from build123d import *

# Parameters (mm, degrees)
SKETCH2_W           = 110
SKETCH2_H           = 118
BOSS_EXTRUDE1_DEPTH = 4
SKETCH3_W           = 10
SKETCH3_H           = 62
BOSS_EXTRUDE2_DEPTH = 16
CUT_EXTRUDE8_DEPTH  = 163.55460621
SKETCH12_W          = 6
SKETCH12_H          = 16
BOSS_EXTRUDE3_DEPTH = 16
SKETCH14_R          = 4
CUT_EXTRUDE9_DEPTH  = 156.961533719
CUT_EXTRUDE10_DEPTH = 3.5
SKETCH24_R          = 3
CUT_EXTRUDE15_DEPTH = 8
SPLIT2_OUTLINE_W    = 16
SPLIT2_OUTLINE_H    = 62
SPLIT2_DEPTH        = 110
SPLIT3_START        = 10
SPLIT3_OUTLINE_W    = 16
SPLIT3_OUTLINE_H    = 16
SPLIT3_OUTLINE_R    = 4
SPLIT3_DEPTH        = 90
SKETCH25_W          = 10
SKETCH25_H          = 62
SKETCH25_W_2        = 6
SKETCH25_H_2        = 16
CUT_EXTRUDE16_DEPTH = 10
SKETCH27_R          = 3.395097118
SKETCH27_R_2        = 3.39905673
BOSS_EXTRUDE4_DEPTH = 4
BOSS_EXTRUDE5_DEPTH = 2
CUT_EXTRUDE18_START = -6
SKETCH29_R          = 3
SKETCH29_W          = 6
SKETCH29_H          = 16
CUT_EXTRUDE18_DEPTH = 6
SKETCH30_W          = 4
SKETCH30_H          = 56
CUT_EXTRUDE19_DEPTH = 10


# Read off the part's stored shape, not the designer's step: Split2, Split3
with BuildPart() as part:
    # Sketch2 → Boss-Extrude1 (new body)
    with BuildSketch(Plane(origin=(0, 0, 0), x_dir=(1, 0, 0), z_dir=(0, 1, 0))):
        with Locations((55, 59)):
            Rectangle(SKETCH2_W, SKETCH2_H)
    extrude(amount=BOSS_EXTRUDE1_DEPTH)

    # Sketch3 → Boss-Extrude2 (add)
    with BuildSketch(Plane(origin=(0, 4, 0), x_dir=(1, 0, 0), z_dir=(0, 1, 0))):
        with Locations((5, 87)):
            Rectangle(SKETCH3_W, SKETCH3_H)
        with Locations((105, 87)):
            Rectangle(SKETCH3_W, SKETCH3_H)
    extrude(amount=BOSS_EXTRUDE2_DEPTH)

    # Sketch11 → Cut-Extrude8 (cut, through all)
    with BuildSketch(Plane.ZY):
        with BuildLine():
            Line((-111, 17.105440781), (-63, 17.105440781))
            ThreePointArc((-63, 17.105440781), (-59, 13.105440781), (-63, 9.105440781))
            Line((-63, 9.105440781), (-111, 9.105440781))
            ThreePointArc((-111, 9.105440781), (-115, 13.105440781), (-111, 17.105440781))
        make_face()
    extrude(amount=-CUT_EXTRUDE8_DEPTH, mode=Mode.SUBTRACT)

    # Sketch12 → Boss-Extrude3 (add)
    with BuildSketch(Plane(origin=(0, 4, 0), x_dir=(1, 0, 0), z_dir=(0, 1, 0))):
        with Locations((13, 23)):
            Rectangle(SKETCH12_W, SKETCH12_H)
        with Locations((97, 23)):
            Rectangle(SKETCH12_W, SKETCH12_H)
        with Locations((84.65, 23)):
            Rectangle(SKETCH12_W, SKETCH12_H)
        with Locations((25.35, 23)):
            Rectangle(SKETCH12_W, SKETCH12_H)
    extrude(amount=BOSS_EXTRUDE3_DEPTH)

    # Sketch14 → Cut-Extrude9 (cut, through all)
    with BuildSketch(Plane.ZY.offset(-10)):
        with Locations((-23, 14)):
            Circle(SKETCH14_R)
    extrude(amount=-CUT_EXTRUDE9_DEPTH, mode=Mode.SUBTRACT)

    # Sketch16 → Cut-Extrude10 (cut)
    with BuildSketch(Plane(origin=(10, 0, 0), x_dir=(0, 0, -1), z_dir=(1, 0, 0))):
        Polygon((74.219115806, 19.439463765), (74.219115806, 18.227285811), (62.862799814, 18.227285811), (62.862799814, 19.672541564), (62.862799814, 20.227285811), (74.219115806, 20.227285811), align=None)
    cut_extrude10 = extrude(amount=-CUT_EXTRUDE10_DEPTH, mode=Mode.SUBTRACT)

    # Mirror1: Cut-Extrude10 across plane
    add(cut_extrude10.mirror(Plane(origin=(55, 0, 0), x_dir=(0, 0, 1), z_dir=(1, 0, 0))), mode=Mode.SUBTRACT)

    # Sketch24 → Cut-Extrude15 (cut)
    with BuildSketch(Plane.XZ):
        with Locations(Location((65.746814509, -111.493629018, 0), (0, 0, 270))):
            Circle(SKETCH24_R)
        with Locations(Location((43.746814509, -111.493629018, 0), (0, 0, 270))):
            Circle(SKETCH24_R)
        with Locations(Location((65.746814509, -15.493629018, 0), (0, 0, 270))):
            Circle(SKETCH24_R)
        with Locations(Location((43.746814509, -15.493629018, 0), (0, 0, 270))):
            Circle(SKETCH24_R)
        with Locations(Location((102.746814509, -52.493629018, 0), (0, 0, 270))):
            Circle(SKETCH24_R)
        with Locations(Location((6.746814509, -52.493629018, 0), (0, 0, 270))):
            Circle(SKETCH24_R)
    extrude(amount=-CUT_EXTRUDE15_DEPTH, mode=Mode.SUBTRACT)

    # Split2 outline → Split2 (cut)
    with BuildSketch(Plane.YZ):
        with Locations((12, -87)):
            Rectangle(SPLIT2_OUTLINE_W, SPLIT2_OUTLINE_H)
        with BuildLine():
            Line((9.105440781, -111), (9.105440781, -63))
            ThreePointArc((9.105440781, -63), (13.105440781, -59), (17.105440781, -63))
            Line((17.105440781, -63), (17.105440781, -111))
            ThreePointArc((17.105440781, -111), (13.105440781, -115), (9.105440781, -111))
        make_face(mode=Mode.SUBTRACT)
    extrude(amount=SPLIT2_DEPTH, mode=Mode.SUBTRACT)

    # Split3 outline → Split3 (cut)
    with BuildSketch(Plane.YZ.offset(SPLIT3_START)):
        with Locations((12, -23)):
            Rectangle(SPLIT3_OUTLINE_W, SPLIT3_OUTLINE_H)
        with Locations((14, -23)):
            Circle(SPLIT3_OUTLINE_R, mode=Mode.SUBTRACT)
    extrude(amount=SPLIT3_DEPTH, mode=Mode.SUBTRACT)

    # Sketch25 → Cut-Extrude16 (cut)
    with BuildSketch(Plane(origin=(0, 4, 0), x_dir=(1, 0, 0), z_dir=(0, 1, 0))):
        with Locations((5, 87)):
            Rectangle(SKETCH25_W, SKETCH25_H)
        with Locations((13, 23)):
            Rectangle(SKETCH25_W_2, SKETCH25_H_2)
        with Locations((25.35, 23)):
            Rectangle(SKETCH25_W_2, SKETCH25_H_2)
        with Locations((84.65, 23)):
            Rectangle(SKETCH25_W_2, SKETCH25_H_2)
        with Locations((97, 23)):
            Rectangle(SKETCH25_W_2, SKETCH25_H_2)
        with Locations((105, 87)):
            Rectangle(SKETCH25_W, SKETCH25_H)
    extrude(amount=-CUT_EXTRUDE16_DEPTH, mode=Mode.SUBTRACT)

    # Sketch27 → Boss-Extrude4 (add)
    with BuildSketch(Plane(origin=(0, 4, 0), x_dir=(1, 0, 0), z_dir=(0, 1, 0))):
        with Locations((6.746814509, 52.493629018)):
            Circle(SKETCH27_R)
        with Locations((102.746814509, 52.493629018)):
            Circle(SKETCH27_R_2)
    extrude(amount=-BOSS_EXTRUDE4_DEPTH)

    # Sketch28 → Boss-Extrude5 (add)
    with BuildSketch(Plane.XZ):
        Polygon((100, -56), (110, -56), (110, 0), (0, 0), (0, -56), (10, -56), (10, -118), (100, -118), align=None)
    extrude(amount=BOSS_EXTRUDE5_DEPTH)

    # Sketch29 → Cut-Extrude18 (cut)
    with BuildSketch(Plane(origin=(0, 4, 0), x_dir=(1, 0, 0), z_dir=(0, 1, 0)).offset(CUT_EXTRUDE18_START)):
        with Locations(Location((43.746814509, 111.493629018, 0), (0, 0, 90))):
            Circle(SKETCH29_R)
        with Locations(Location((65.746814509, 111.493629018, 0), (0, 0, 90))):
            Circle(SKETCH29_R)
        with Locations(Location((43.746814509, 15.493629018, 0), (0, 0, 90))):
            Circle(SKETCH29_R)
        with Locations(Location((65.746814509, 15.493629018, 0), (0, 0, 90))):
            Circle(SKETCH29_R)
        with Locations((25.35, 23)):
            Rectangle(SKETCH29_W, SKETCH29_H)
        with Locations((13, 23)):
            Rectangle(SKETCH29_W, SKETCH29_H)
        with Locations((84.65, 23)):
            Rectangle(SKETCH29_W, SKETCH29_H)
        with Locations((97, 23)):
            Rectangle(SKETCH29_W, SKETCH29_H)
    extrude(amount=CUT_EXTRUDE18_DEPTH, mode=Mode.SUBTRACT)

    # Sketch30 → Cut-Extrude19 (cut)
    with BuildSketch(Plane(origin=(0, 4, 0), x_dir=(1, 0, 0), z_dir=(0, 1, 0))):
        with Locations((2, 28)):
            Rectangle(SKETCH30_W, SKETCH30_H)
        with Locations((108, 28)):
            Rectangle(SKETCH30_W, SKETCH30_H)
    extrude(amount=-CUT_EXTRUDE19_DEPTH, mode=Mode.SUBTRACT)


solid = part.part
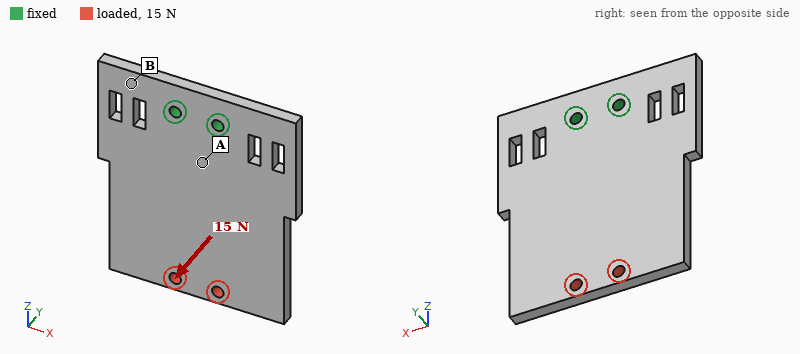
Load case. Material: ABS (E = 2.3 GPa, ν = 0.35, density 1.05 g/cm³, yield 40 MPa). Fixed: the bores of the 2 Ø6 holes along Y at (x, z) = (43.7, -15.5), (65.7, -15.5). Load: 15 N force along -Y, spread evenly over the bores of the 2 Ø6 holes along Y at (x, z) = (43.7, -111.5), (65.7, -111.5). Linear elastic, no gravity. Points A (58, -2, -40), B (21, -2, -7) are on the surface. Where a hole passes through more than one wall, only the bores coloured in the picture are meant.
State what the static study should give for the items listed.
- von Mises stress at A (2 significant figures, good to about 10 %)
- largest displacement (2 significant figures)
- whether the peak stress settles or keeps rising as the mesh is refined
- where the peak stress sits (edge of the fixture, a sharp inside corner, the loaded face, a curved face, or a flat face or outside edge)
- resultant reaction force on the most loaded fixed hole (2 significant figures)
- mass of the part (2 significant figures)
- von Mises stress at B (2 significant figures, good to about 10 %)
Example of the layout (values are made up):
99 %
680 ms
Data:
2.0 MPa
1.5 mm
keeps rising
edge of the fixture
7.5 N
68 g
0.75 MPa
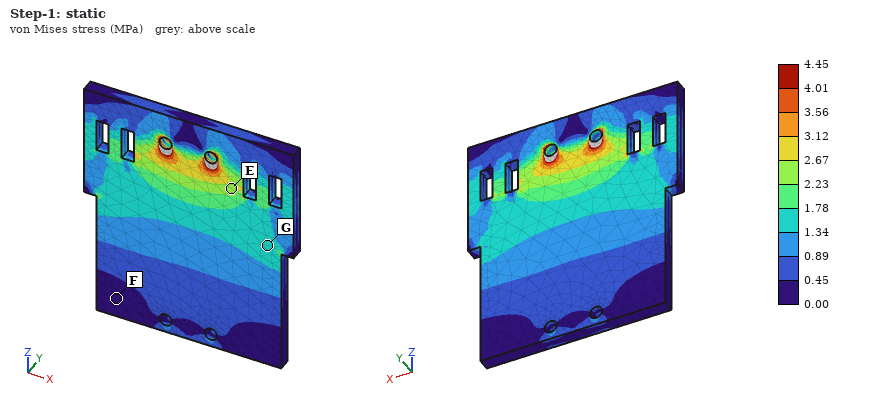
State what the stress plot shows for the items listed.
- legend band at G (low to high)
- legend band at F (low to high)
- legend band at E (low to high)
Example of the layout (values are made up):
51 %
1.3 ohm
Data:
1.34 to 1.78 MPa
0.00 to 0.45 MPa
2.23 to 2.67 MPa
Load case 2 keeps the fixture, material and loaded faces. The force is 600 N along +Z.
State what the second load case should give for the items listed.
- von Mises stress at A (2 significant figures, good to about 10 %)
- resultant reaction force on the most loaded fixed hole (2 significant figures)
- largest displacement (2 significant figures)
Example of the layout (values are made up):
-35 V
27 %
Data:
1.9 MPa
300 N
92 µm
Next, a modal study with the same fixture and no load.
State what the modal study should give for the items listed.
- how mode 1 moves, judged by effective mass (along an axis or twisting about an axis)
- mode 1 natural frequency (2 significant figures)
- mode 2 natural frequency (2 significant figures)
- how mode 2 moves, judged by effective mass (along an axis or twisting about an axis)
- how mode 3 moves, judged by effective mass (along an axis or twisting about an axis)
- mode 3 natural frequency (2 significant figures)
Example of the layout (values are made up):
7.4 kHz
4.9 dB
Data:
along Y
130 Hz
300 Hz
twisting about Z
along X
660 Hz
